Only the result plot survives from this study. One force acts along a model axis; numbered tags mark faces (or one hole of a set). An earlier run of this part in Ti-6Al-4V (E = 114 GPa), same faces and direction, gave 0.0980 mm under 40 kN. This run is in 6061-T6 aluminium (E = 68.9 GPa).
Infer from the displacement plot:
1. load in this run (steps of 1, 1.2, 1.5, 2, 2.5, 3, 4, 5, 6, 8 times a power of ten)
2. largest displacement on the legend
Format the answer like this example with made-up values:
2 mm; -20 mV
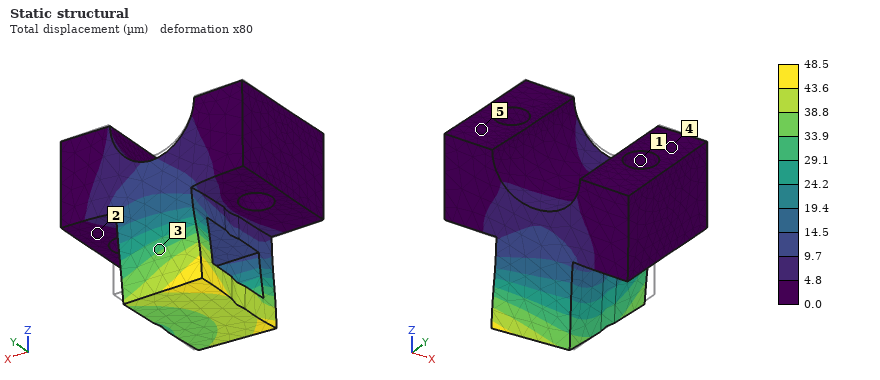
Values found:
12 kN; 48.5 µm
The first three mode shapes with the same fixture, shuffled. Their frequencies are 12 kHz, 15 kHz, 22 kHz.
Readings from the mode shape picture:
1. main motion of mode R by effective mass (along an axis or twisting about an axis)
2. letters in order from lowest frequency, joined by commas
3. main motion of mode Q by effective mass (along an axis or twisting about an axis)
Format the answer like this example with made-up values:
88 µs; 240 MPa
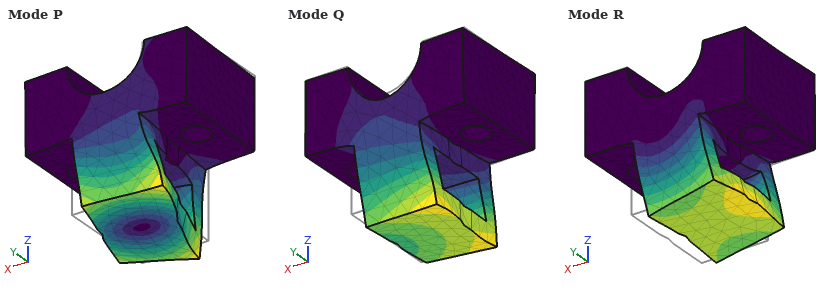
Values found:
along X; Q, R, P; along Y
